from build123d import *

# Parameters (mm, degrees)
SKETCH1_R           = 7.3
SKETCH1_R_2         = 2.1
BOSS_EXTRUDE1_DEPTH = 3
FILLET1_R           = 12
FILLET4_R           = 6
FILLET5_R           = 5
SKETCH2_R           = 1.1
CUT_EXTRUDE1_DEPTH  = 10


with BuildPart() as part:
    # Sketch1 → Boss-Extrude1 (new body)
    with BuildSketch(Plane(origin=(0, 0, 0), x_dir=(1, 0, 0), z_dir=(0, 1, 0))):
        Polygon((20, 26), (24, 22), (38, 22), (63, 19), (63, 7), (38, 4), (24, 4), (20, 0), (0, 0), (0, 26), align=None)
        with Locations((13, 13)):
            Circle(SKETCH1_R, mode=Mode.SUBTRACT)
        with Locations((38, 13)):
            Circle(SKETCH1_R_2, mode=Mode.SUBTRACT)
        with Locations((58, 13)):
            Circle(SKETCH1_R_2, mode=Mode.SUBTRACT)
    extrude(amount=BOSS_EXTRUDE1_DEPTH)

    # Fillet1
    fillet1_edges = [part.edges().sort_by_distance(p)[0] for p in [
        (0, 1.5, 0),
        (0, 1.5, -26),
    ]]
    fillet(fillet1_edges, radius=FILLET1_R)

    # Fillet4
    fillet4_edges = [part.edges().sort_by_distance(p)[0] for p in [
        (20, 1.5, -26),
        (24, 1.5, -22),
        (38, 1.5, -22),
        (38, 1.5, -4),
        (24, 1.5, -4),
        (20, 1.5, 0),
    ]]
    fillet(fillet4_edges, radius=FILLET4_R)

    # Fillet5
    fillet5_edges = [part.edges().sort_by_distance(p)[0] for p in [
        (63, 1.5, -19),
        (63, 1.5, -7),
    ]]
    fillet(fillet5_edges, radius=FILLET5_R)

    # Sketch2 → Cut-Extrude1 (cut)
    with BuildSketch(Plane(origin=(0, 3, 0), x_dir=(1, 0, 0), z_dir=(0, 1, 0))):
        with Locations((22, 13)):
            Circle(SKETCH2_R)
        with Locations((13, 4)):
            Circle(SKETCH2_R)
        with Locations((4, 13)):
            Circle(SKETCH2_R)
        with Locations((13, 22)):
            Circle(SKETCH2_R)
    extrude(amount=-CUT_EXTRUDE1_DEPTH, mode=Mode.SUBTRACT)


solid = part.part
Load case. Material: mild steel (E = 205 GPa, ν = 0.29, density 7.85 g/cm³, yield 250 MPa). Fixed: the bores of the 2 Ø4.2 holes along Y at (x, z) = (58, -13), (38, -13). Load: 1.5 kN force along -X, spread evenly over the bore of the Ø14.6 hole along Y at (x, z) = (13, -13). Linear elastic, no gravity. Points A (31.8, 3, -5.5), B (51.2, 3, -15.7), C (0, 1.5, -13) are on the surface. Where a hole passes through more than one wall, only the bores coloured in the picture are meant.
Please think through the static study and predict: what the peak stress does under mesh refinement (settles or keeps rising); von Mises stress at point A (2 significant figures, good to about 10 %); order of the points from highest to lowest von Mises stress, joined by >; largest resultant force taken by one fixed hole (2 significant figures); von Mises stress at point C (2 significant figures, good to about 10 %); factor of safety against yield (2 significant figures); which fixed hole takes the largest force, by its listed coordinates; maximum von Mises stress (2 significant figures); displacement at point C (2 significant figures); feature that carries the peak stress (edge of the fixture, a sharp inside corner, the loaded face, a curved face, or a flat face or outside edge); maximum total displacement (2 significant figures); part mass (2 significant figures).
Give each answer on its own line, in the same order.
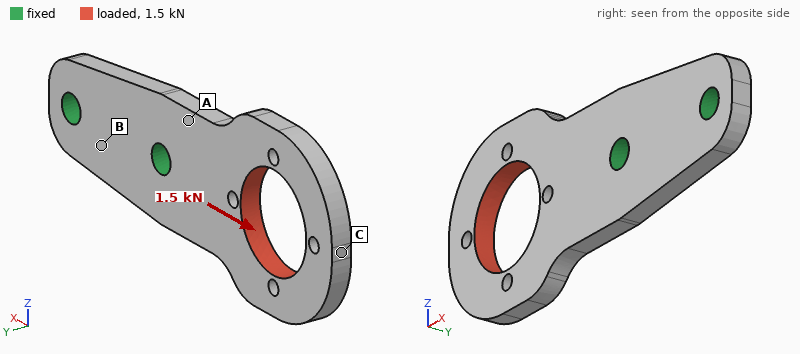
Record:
settles
28 MPa
C > A > B
1.3 kN
48 MPa
1.1
(38, -13)
230 MPa
10.0 µm
a curved face
11 µm
22 g
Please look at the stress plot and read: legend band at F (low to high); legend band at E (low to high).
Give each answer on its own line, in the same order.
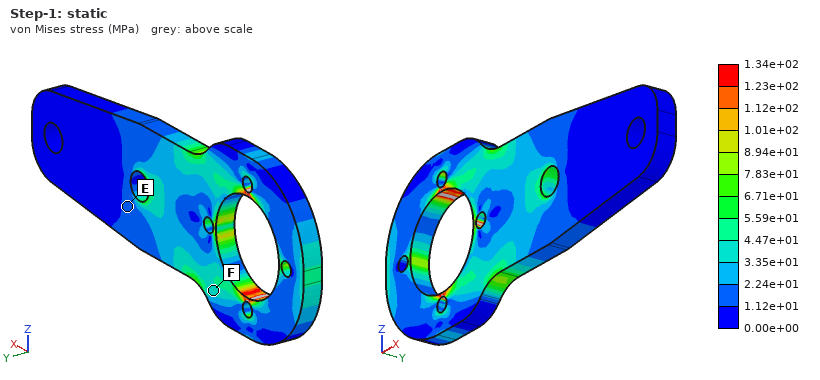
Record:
3.35e+01 to 4.47e+01 MPa
1.12e+01 to 2.24e+01 MPa
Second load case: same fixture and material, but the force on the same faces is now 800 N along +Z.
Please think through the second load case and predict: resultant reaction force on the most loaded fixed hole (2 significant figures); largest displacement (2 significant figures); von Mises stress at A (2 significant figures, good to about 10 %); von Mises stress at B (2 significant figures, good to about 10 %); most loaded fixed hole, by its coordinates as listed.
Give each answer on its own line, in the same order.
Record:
1.4 kN
65 µm
80 MPa
32 MPa
(38, -13)
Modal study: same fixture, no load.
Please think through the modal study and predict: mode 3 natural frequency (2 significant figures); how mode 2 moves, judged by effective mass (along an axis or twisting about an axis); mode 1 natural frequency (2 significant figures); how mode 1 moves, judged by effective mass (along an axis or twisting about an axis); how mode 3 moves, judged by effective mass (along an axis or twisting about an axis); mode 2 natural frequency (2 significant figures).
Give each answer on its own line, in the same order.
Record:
6600 Hz
twisting about X
1900 Hz
along Y
along Z
4700 Hz
